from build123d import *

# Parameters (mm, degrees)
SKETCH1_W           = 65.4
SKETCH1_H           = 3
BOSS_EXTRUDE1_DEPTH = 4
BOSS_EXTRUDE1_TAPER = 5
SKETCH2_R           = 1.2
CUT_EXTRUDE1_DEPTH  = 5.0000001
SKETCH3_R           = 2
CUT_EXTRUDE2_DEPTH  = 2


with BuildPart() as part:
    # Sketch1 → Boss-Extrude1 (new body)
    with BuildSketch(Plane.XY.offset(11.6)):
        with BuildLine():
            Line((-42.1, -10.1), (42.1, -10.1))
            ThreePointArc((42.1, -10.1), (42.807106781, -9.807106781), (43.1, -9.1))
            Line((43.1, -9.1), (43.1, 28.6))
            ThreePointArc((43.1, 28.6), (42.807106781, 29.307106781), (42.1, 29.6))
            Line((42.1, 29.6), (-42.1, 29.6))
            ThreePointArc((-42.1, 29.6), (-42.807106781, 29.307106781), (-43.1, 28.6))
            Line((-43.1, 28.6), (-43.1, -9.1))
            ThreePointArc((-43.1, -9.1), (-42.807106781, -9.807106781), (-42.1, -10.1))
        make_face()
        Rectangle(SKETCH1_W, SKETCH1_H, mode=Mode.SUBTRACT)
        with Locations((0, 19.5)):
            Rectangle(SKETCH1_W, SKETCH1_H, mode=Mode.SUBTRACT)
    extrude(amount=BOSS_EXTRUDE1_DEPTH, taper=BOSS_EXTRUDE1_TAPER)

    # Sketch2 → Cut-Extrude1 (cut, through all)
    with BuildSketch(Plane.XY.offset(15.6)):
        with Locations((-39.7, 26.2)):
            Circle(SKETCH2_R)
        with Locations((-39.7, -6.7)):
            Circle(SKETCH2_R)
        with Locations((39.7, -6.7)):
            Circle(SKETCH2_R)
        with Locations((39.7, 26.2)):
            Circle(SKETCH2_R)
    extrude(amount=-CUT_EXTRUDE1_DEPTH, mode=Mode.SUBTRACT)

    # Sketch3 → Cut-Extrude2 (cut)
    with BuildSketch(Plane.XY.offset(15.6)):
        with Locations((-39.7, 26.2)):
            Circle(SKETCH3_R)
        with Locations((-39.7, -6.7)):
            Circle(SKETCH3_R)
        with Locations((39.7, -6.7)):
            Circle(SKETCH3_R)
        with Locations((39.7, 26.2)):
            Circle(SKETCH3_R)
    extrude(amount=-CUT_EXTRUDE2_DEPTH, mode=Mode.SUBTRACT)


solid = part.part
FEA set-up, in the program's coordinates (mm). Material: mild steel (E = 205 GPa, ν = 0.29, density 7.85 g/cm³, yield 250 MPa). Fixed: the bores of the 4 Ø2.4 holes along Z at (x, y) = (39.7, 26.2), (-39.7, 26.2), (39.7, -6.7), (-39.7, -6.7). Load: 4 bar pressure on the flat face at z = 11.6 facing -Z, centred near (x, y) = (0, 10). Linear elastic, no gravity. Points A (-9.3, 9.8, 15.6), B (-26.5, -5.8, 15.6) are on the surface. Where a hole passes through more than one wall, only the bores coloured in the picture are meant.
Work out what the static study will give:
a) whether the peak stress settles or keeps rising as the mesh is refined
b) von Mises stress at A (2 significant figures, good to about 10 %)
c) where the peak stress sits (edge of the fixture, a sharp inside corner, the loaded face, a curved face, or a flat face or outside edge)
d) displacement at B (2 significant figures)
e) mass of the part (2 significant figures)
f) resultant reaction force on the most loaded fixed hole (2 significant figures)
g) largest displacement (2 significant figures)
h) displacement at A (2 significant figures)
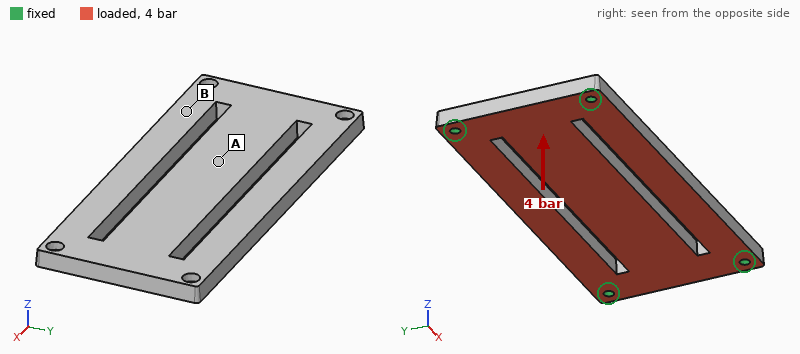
keeps rising
57 MPa
edge of the fixture
29 µm
91 g
510 N
84 µm
77 µm
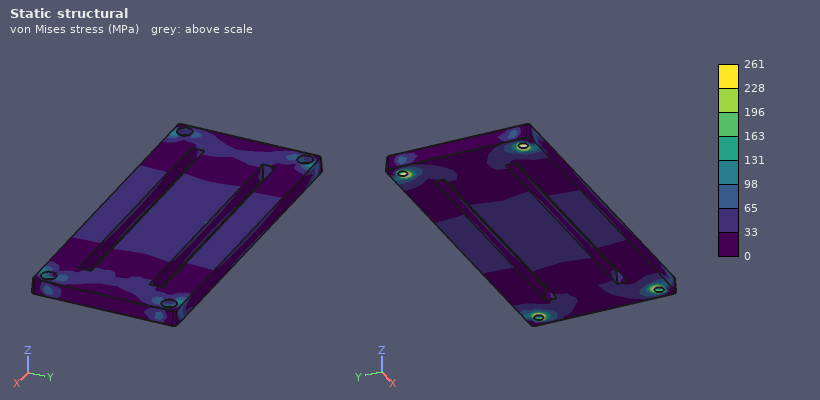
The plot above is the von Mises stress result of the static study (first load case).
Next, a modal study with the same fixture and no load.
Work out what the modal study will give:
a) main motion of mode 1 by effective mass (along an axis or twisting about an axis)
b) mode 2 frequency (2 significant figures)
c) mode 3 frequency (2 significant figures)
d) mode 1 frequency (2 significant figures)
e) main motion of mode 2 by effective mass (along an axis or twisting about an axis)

along Z
3200 Hz
3500 Hz
2300 Hz
twisting about X
